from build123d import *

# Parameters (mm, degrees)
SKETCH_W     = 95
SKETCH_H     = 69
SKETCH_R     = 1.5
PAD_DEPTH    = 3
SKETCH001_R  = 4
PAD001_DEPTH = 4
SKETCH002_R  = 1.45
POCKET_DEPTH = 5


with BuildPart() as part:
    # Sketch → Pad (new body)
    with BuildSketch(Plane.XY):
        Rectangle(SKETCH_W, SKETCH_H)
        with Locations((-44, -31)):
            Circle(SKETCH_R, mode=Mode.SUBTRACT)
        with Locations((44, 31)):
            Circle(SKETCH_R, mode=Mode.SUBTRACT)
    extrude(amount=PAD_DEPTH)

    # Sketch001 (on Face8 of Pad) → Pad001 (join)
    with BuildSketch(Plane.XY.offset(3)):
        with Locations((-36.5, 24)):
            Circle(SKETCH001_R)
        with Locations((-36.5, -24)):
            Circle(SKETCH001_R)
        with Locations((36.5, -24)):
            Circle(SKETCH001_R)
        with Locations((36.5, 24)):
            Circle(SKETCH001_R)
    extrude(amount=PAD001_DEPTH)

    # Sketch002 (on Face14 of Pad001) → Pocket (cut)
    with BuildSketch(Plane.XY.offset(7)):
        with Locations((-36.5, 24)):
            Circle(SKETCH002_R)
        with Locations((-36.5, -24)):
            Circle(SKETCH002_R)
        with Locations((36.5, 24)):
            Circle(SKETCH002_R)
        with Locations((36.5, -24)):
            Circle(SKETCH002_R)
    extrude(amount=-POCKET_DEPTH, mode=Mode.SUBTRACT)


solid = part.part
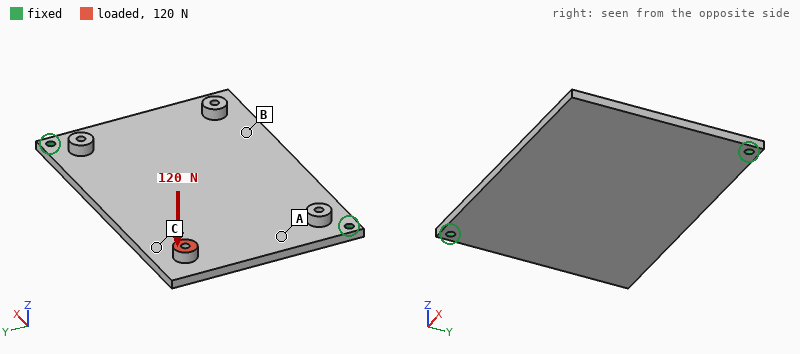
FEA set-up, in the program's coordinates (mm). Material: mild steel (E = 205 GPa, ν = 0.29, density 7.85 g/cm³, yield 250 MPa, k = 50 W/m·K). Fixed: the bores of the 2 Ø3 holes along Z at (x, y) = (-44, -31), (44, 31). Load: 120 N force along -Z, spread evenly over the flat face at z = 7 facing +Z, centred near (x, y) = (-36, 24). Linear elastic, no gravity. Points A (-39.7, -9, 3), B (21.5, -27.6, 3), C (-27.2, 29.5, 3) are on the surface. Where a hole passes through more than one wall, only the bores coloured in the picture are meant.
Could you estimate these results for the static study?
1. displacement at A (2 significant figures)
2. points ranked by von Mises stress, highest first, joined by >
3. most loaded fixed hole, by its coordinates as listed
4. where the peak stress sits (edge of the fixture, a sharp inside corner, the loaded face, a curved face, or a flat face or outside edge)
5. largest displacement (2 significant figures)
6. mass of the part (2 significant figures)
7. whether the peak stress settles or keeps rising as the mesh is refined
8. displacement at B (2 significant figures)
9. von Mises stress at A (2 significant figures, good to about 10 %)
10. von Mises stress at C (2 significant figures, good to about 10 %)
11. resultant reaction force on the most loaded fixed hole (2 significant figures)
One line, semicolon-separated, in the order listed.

0.072 mm; A > C > B; (-44, -31); edge of the fixture; 0.35 mm; 160 g; keeps rising; 0.084 mm; 44 MPa; 28 MPa; 81 N
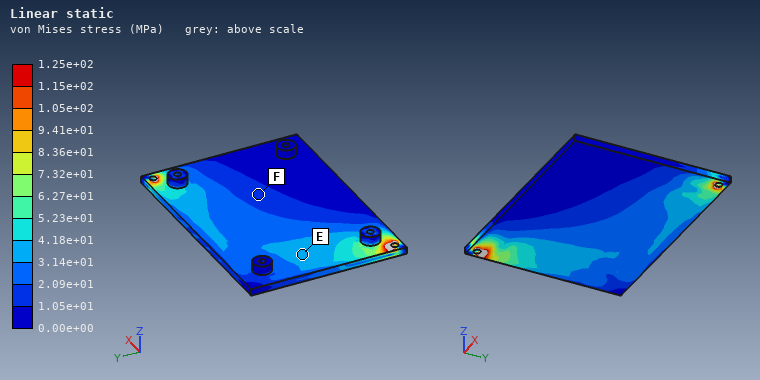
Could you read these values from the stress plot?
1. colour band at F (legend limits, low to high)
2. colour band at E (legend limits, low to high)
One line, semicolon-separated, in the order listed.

1.05e+01 to 2.09e+01 MPa; 3.14e+01 to 4.18e+01 MPa
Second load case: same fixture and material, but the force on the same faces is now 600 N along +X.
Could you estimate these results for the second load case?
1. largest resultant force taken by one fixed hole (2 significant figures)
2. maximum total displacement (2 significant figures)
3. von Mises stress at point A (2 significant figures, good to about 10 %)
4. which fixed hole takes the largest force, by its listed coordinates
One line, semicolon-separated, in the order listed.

390 N; 0.16 mm; 34 MPa; (44, 31)
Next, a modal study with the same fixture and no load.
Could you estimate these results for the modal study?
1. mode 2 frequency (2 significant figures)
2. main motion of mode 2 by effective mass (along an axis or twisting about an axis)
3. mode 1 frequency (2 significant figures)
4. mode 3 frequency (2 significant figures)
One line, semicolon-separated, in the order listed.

780 Hz; along Z; 610 Hz; 2000 Hz
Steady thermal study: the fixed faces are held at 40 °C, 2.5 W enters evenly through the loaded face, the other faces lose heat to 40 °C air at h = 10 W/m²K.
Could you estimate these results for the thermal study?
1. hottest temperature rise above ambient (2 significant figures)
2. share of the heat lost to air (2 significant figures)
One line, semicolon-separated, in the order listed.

24 K; 39 %
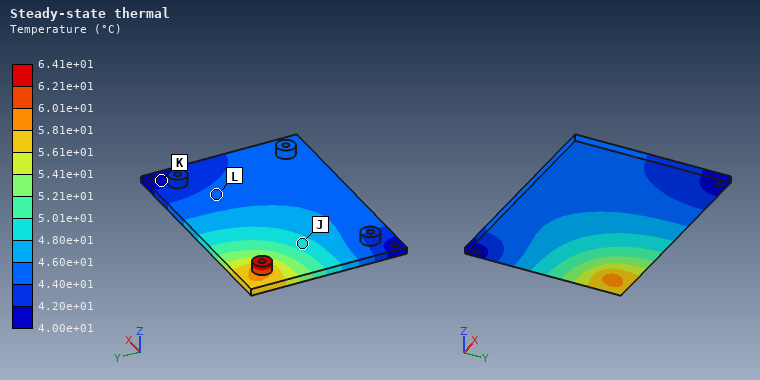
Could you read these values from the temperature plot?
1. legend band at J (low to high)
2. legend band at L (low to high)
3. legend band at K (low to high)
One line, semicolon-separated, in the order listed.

4.80e+01 to 5.01e+01 °C; 4.40e+01 to 4.60e+01 °C; 4.00e+01 to 4.20e+01 °C
